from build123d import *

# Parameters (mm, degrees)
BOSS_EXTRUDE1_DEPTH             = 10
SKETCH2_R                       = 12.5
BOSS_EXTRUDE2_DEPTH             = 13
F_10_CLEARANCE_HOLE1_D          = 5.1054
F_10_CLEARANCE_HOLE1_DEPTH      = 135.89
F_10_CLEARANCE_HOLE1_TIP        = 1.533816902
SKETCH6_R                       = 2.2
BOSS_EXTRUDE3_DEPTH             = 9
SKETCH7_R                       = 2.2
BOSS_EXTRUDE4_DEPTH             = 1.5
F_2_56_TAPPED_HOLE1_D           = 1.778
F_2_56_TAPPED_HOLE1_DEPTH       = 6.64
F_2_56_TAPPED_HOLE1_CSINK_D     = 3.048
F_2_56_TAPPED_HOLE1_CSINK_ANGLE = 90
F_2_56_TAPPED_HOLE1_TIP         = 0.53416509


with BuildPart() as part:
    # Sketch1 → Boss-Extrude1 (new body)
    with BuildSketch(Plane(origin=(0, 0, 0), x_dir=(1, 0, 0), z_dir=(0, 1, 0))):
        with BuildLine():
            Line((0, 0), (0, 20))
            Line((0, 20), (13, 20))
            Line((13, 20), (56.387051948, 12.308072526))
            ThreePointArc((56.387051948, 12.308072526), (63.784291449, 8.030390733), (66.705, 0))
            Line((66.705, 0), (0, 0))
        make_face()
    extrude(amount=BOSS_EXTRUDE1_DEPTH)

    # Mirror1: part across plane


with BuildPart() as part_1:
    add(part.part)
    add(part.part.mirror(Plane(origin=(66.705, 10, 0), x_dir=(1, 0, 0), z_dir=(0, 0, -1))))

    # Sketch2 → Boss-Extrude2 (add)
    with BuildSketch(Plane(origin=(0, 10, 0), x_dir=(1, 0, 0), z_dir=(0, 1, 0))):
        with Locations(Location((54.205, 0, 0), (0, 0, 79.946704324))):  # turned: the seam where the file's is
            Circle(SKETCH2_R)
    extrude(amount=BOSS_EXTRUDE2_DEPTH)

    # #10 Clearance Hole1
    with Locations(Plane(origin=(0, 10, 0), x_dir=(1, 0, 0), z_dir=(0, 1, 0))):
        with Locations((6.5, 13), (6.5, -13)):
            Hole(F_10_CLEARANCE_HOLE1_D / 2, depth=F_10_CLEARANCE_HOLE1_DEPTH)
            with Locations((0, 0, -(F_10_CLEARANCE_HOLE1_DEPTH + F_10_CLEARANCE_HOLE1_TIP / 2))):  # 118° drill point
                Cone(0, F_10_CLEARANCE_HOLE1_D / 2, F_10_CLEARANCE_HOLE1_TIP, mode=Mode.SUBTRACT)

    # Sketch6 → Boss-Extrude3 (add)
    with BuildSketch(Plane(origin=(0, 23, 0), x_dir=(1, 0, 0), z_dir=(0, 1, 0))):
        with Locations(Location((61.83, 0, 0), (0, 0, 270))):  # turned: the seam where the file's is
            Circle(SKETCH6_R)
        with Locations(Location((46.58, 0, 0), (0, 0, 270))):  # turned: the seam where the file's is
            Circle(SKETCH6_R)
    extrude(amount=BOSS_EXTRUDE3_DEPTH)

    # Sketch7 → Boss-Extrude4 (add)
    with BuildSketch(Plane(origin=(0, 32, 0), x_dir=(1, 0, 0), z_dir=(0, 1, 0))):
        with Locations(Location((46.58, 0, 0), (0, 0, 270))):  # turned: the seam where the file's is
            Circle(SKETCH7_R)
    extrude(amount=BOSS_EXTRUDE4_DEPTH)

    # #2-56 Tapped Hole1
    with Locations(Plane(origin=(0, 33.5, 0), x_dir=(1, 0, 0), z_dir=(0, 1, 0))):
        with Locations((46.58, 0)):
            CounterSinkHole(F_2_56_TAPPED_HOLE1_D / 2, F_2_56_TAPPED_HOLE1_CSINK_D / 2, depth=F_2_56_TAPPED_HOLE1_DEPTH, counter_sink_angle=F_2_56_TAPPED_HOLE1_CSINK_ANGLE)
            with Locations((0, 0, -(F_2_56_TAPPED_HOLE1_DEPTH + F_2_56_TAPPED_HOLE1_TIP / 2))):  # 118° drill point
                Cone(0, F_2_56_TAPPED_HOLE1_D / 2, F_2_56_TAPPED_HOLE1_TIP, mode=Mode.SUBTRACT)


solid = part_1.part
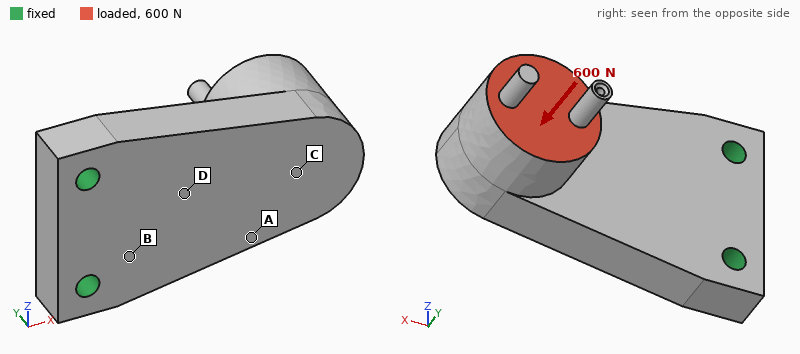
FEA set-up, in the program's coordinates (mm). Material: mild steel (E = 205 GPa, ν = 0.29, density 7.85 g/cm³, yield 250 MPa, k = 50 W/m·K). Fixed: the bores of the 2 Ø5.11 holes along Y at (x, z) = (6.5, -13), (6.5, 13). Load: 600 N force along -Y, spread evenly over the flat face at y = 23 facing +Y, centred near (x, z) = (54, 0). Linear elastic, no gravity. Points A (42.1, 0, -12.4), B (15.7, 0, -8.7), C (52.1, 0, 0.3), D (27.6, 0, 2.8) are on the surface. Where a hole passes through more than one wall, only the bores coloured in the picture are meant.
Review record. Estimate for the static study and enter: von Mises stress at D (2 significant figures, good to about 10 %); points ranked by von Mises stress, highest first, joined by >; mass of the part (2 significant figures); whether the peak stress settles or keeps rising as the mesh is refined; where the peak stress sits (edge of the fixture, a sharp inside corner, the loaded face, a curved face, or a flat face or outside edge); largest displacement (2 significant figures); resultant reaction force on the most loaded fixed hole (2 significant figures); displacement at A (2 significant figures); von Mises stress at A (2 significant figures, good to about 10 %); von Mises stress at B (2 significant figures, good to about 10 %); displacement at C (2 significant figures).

27 MPa
B > D > A > C
210 g
keeps rising
edge of the fixture
58 µm
300 N
24 µm
14 MPa
35 MPa
35 µm
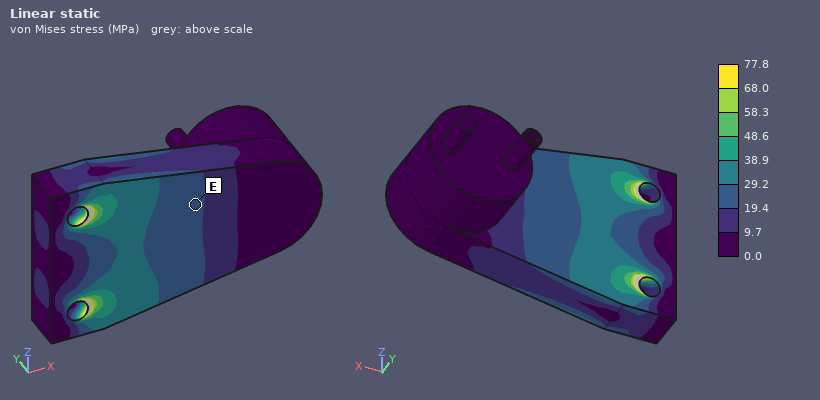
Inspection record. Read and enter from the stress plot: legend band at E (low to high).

19.4 to 29.2 MPa
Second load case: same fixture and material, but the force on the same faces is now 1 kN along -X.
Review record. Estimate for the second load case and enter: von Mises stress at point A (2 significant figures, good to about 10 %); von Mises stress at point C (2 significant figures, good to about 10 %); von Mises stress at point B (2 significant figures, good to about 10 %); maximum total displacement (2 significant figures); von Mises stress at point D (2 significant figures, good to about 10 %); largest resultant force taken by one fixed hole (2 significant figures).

29 MPa
10 MPa
25 MPa
60 µm
27 MPa
510 N
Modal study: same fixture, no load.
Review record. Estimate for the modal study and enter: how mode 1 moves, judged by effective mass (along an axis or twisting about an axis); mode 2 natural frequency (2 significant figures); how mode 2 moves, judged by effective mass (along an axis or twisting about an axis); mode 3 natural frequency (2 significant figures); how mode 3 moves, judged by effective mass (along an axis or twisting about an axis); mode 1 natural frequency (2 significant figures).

along Y
5200 Hz
along Z
8600 Hz
along Z
1900 Hz
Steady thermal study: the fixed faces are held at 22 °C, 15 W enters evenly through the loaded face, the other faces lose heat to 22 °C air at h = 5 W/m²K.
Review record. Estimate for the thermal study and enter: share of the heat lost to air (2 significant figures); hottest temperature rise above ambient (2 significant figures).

5.0 %
47 K
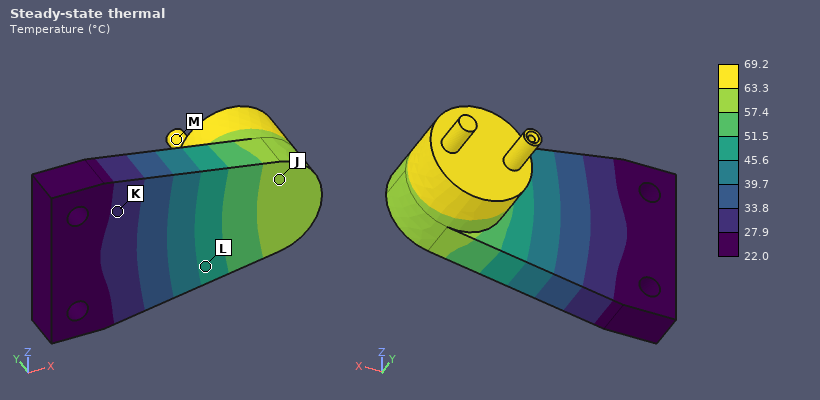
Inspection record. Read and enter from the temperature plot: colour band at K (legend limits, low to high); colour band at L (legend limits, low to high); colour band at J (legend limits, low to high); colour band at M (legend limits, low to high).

27.9 to 33.8 °C
45.6 to 51.5 °C
57.4 to 63.3 °C
63.3 to 69.2 °C
